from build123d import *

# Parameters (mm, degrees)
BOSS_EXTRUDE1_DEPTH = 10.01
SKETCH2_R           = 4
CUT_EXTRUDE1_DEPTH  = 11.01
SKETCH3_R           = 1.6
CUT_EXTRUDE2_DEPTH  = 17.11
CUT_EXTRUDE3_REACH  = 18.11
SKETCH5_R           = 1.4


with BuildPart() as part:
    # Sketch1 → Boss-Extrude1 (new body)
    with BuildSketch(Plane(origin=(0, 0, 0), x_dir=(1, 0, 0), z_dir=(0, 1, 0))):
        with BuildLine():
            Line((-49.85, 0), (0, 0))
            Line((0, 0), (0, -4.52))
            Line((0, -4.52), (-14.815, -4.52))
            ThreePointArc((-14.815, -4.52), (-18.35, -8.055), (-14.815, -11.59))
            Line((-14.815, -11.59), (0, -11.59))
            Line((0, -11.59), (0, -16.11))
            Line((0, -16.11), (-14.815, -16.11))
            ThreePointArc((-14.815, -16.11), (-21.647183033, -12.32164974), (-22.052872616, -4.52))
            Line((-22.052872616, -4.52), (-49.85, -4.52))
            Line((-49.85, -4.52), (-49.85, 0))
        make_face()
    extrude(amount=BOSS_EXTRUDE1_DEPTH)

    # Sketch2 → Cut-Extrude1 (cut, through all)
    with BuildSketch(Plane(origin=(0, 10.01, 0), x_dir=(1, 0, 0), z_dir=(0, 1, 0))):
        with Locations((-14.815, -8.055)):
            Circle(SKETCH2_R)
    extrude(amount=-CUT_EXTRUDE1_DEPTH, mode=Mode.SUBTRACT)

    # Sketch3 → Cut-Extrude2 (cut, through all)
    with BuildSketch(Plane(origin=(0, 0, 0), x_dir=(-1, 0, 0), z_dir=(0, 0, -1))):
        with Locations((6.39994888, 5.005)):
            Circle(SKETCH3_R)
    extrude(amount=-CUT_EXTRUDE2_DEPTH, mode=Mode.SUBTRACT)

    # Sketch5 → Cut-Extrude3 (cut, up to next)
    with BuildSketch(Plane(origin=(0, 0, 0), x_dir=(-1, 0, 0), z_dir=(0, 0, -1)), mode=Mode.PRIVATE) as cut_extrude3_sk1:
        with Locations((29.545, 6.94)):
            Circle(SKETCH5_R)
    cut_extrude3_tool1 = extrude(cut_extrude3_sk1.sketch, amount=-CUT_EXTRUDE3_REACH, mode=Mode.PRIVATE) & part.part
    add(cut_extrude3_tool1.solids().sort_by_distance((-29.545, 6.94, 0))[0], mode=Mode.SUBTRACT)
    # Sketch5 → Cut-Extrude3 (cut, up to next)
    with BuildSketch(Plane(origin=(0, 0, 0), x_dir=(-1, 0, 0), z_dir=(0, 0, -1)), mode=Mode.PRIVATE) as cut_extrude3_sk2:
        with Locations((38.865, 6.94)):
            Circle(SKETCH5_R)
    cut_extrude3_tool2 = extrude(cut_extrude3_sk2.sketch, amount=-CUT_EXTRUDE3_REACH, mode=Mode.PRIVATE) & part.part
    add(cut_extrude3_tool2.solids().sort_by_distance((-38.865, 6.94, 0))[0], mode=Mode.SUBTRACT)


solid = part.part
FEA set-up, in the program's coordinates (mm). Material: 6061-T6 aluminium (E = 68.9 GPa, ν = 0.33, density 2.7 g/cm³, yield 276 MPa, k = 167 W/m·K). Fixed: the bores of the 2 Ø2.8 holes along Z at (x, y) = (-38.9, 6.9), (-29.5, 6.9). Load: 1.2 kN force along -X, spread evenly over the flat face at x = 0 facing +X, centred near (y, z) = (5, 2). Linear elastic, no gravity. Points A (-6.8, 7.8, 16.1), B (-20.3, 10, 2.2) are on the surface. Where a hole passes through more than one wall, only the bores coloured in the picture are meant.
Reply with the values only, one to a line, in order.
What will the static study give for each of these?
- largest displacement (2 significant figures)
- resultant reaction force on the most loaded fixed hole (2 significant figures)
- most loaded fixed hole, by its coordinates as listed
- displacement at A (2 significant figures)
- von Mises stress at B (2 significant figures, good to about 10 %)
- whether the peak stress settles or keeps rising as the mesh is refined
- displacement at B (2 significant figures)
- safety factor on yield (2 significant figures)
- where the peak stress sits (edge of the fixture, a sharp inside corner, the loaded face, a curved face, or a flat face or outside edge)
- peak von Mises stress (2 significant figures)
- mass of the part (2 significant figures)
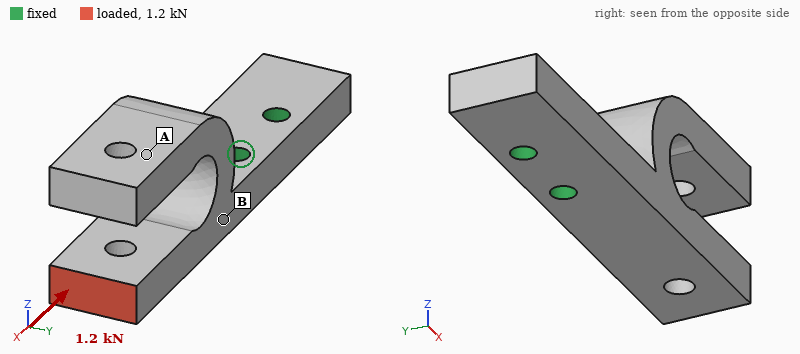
19 µm
990 N
(-29.5, 6.9)
8.9 µm
28 MPa
settles
3.6 µm
3.0
a curved face
92 MPa
9.0 g
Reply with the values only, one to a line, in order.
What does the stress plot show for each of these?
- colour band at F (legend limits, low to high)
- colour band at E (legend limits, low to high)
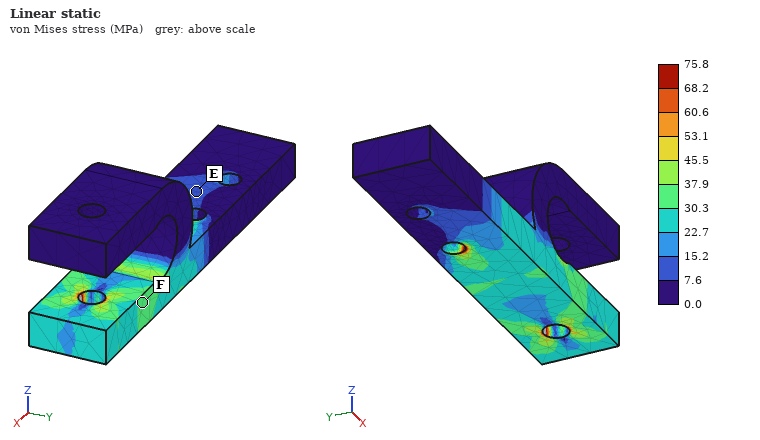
30.3 to 37.9 MPa
7.6 to 15.2 MPa
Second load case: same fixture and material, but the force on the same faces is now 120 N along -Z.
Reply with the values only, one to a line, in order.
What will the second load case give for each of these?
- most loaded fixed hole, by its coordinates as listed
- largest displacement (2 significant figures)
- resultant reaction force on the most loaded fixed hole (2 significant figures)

(-29.5, 6.9)
0.19 mm
210 N
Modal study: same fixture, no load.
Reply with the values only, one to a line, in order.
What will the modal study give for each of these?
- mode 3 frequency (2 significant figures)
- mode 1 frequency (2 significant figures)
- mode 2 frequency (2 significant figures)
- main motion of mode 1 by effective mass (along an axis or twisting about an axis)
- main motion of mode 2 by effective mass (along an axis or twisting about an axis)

6500 Hz
2600 Hz
4200 Hz
along Z
along Y
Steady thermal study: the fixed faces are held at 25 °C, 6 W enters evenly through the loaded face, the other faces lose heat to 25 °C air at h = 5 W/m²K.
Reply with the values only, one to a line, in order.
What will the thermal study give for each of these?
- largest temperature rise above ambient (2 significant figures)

24 K
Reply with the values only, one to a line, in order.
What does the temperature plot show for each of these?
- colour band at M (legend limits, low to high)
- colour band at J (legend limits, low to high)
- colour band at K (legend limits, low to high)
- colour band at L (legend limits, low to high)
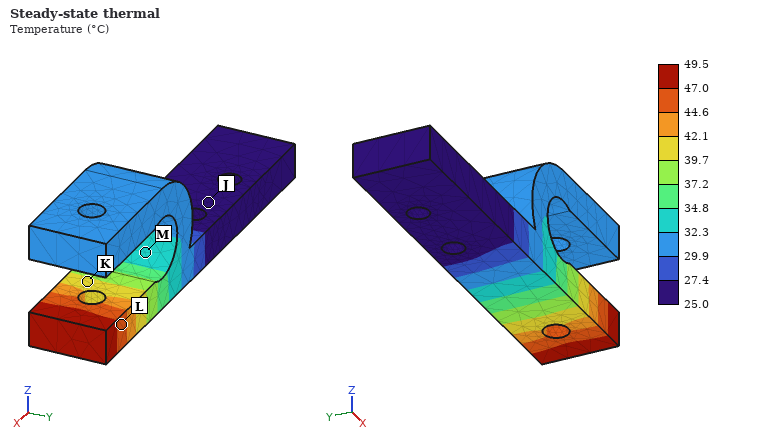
32.3 to 34.8 °C
25.0 to 27.4 °C
39.7 to 42.1 °C
44.6 to 47.0 °C
